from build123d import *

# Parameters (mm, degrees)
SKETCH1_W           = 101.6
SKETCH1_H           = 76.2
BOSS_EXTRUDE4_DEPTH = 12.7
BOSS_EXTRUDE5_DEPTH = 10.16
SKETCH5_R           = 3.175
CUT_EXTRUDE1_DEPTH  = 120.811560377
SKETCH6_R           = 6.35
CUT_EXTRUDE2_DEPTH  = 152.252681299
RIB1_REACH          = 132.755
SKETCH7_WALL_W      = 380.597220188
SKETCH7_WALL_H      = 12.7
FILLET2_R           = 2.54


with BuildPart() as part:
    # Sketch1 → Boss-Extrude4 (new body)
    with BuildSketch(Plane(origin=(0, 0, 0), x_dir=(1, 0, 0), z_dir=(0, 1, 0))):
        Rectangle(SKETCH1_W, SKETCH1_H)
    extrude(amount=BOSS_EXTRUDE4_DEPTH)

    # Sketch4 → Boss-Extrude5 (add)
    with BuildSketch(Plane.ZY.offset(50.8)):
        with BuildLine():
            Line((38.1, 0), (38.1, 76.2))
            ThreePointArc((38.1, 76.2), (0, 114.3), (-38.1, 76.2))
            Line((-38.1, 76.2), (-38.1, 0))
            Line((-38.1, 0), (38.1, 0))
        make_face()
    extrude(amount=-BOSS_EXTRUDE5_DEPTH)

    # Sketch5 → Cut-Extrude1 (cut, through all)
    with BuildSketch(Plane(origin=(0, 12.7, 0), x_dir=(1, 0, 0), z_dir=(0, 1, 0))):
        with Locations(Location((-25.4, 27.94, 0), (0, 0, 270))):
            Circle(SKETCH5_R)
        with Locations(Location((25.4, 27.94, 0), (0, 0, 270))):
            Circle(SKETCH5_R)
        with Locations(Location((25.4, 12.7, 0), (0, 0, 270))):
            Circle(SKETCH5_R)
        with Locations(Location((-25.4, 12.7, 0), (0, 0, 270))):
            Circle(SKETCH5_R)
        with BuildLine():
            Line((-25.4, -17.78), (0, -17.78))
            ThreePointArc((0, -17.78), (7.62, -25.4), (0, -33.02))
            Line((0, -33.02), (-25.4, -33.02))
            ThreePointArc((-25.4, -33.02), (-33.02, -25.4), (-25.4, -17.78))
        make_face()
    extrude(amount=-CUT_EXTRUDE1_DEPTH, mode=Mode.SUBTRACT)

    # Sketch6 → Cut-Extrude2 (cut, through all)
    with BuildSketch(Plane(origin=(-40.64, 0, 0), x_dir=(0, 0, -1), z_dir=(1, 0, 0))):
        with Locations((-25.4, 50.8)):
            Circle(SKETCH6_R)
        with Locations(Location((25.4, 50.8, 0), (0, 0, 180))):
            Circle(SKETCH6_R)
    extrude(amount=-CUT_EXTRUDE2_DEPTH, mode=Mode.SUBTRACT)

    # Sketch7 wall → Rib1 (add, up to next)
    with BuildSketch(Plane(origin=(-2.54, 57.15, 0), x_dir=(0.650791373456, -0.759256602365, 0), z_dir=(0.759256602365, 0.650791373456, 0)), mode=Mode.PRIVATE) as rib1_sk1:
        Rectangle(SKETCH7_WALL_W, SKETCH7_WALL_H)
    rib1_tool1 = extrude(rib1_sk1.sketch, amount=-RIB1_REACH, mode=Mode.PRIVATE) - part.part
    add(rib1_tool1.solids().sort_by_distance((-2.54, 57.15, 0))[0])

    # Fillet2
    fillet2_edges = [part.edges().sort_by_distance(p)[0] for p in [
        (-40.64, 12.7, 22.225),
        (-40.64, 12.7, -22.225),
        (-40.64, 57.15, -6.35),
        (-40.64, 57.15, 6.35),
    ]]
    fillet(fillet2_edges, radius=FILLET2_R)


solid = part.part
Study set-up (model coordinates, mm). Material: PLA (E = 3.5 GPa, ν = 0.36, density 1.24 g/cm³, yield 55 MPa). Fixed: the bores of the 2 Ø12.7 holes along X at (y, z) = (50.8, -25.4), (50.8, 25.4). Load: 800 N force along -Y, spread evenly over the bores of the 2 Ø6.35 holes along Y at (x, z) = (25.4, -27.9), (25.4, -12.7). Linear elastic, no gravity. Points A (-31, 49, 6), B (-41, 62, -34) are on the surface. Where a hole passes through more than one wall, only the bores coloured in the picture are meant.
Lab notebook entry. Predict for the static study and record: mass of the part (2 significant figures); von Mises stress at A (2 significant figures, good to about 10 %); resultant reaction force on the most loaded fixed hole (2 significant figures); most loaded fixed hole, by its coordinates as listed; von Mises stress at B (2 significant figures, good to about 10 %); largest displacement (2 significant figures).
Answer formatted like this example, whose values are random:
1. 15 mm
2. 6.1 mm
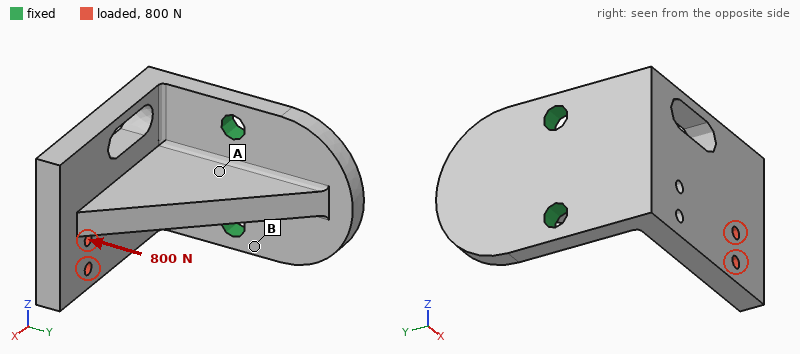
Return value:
1. 250 g
2. 4.4 MPa
3. 690 N
4. (50.8, -25.4)
5. 11 MPa
6. 2.0 mm
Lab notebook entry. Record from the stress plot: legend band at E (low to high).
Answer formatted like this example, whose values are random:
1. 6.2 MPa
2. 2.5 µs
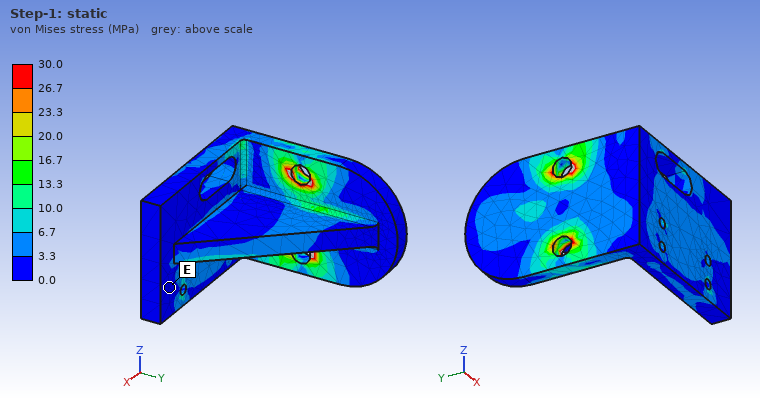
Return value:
1. 0.0 to 3.3 MPa
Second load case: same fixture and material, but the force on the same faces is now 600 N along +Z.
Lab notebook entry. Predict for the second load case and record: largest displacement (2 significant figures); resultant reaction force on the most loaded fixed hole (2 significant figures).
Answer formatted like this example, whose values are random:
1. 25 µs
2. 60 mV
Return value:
1. 1.3 mm
2. 1.1 kN
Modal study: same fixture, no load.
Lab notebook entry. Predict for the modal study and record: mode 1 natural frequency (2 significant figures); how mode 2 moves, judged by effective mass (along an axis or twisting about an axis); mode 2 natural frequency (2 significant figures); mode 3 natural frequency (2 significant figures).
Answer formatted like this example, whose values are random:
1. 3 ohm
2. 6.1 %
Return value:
1. 390 Hz
2. along Z
3. 450 Hz
4. 1100 Hz
